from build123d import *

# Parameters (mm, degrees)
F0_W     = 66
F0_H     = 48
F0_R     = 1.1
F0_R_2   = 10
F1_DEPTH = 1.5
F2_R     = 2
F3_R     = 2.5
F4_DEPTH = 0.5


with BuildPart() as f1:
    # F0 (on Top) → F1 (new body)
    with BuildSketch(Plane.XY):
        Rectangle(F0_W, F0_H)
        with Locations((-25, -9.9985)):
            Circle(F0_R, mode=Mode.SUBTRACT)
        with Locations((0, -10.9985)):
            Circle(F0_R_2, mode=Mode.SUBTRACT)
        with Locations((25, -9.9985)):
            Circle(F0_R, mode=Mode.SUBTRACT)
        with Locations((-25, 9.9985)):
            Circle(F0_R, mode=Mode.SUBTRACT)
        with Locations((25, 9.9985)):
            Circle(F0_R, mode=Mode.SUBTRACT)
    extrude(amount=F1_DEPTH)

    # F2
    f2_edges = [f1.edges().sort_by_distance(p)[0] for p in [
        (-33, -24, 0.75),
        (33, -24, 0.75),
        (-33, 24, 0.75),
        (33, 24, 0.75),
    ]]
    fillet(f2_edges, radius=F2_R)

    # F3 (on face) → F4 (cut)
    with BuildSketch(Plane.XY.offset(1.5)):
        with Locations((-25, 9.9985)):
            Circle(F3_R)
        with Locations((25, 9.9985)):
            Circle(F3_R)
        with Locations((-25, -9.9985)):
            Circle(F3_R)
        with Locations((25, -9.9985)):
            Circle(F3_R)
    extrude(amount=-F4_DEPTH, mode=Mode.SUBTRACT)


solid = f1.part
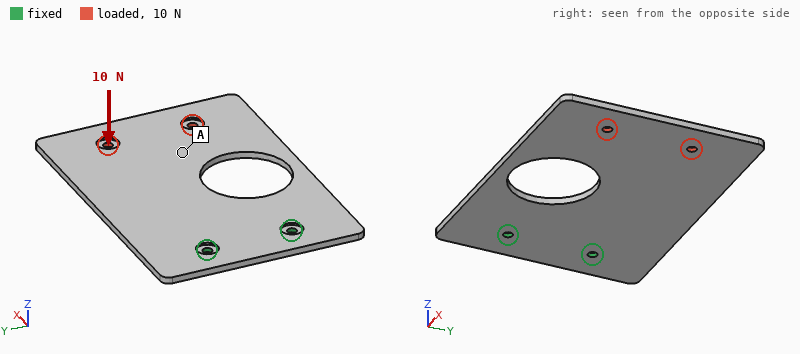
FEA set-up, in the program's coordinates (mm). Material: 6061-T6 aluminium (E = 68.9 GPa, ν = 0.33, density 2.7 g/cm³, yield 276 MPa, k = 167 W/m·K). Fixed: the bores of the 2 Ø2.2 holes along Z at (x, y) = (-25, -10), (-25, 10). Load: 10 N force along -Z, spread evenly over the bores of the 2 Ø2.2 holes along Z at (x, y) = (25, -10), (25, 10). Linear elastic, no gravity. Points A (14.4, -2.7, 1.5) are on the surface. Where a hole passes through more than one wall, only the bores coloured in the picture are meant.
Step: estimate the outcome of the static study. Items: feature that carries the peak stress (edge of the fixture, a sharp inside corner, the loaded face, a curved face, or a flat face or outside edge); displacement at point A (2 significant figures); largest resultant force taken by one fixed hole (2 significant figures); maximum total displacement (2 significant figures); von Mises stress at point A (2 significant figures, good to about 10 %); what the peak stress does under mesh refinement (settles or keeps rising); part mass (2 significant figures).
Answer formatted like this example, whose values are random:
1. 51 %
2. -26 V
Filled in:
1. edge of the fixture
2. 0.47 mm
3. 9.9 N
4. 0.84 mm
5. 6.7 MPa
6. keeps rising
7. 11 g
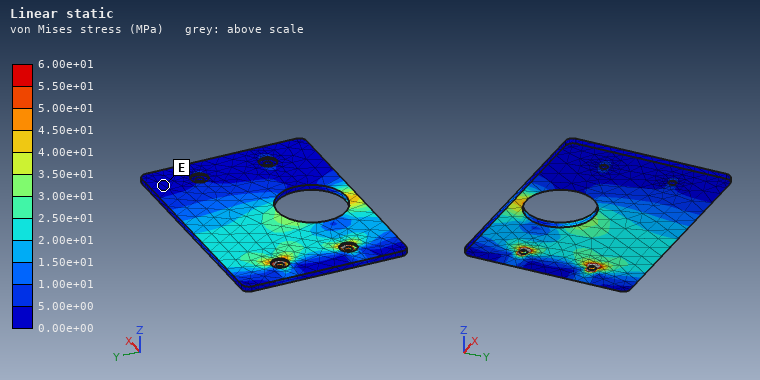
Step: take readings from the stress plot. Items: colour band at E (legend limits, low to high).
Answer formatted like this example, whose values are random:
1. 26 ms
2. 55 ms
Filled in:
1. 0.00e+00 to 5.00e+00 MPa
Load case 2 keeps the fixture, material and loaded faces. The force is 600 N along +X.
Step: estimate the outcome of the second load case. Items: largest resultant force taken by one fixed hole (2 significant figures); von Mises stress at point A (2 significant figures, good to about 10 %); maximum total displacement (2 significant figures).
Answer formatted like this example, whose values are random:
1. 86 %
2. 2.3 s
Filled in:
1. 300 N
2. 7.6 MPa
3. 0.33 mm
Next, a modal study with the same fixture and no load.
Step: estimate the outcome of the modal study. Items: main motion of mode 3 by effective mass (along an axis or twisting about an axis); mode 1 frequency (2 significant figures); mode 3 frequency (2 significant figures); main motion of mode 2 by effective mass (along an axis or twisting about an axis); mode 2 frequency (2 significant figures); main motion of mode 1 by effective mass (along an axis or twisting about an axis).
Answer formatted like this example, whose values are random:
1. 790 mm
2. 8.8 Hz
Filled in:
1. along Z
2. 300 Hz
3. 2000 Hz
4. twisting about X
5. 870 Hz
6. along Z
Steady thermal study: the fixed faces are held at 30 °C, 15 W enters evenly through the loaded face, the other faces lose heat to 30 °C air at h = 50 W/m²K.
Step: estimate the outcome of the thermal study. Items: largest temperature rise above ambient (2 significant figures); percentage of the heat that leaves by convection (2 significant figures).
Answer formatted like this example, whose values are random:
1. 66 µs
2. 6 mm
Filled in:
1. 63 K
2. 55 %
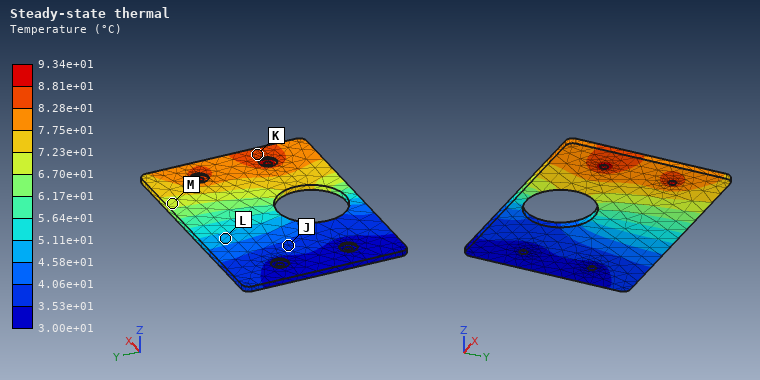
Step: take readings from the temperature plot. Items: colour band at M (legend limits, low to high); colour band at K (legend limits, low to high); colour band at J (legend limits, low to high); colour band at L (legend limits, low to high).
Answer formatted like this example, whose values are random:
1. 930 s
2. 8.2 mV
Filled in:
1. 6.70e+01 to 7.23e+01 °C
2. 8.28e+01 to 8.81e+01 °C
3. 3.53e+01 to 4.06e+01 °C
4. 4.58e+01 to 5.11e+01 °C
